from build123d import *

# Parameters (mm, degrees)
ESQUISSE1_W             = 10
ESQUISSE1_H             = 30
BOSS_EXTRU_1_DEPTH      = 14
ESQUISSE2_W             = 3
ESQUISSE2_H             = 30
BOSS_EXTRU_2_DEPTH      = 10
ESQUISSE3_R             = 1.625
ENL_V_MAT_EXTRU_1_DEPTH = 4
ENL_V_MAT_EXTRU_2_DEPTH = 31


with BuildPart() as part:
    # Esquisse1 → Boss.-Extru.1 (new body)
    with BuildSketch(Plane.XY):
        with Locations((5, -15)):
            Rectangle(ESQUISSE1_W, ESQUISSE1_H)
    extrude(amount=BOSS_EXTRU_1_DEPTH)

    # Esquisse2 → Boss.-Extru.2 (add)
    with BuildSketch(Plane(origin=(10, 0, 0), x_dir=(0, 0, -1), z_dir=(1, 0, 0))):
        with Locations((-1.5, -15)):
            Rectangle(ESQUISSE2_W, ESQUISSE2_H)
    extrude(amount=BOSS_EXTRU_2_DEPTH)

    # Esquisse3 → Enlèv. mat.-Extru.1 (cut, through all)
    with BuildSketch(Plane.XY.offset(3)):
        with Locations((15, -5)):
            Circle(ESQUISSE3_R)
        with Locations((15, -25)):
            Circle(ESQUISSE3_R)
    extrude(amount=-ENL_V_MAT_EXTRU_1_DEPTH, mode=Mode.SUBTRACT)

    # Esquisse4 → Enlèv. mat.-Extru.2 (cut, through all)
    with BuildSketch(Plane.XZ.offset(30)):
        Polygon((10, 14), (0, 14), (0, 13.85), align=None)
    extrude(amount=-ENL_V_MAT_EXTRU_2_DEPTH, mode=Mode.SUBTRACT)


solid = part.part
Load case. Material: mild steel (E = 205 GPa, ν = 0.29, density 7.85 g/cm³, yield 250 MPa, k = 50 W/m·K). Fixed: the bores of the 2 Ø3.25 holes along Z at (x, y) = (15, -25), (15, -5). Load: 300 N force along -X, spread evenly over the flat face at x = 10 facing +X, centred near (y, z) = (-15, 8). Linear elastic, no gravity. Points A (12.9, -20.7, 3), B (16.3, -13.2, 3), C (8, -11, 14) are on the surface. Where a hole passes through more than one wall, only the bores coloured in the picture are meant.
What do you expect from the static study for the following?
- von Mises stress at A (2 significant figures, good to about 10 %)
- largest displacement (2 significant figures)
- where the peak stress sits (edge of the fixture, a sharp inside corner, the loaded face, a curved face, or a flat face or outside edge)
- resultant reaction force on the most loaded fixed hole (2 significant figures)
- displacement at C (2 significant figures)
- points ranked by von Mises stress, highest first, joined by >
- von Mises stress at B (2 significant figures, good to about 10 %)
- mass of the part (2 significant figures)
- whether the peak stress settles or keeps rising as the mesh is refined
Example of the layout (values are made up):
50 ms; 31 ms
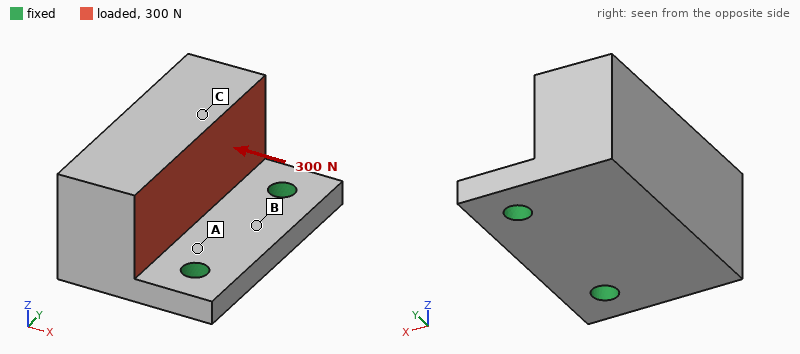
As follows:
34 MPa; 17 µm; edge of the fixture; 150 N; 13 µm; A > B > C; 12 MPa; 39 g; keeps rising
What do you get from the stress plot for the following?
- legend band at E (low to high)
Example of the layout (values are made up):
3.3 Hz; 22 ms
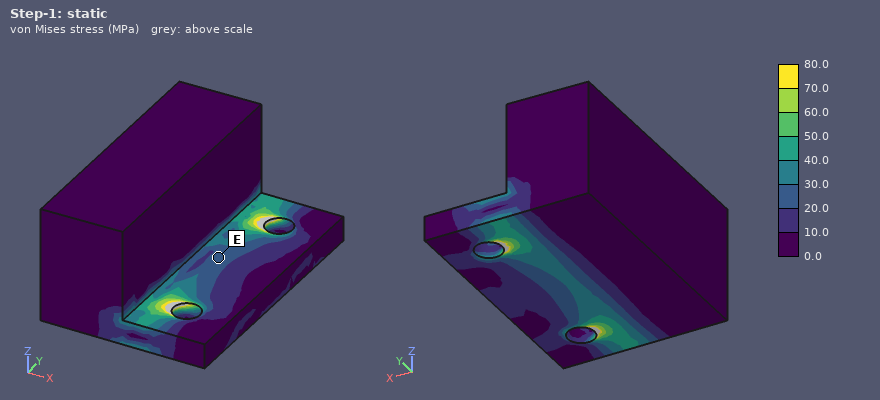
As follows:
20.0 to 30.0 MPa
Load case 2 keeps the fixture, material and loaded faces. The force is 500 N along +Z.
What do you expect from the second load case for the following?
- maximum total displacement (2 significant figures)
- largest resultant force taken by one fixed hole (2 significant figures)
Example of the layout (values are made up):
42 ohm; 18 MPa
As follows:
7.9 µm; 250 N
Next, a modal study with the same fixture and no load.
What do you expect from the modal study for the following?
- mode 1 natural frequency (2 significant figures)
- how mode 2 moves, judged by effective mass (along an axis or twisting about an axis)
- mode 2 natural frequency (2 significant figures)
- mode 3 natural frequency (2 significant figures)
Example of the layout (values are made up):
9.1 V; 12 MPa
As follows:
4000 Hz; along Y; 13 kHz; 21 kHz
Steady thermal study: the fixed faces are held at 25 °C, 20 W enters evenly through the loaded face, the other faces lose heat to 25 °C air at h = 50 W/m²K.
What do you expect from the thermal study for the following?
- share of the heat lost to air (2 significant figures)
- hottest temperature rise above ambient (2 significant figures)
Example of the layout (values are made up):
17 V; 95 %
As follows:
13 %; 42 K
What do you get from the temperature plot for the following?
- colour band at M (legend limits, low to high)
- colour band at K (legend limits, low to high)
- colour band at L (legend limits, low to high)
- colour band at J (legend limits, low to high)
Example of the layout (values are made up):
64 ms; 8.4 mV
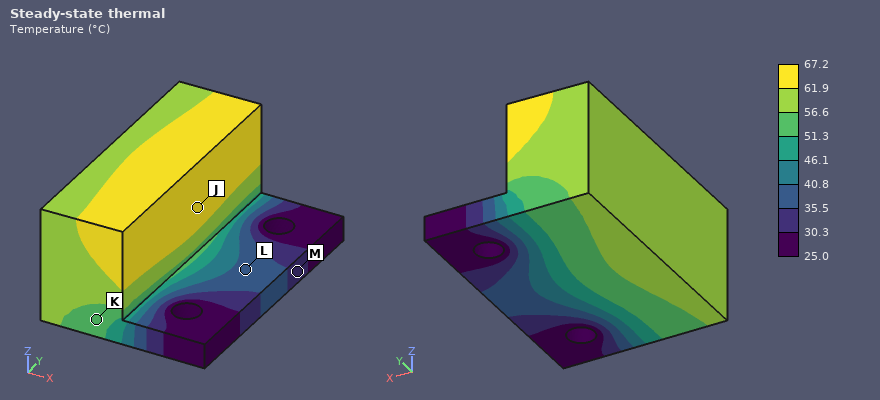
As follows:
30.3 to 35.5 °C; 51.3 to 56.6 °C; 35.5 to 40.8 °C; 61.9 to 67.2 °C
